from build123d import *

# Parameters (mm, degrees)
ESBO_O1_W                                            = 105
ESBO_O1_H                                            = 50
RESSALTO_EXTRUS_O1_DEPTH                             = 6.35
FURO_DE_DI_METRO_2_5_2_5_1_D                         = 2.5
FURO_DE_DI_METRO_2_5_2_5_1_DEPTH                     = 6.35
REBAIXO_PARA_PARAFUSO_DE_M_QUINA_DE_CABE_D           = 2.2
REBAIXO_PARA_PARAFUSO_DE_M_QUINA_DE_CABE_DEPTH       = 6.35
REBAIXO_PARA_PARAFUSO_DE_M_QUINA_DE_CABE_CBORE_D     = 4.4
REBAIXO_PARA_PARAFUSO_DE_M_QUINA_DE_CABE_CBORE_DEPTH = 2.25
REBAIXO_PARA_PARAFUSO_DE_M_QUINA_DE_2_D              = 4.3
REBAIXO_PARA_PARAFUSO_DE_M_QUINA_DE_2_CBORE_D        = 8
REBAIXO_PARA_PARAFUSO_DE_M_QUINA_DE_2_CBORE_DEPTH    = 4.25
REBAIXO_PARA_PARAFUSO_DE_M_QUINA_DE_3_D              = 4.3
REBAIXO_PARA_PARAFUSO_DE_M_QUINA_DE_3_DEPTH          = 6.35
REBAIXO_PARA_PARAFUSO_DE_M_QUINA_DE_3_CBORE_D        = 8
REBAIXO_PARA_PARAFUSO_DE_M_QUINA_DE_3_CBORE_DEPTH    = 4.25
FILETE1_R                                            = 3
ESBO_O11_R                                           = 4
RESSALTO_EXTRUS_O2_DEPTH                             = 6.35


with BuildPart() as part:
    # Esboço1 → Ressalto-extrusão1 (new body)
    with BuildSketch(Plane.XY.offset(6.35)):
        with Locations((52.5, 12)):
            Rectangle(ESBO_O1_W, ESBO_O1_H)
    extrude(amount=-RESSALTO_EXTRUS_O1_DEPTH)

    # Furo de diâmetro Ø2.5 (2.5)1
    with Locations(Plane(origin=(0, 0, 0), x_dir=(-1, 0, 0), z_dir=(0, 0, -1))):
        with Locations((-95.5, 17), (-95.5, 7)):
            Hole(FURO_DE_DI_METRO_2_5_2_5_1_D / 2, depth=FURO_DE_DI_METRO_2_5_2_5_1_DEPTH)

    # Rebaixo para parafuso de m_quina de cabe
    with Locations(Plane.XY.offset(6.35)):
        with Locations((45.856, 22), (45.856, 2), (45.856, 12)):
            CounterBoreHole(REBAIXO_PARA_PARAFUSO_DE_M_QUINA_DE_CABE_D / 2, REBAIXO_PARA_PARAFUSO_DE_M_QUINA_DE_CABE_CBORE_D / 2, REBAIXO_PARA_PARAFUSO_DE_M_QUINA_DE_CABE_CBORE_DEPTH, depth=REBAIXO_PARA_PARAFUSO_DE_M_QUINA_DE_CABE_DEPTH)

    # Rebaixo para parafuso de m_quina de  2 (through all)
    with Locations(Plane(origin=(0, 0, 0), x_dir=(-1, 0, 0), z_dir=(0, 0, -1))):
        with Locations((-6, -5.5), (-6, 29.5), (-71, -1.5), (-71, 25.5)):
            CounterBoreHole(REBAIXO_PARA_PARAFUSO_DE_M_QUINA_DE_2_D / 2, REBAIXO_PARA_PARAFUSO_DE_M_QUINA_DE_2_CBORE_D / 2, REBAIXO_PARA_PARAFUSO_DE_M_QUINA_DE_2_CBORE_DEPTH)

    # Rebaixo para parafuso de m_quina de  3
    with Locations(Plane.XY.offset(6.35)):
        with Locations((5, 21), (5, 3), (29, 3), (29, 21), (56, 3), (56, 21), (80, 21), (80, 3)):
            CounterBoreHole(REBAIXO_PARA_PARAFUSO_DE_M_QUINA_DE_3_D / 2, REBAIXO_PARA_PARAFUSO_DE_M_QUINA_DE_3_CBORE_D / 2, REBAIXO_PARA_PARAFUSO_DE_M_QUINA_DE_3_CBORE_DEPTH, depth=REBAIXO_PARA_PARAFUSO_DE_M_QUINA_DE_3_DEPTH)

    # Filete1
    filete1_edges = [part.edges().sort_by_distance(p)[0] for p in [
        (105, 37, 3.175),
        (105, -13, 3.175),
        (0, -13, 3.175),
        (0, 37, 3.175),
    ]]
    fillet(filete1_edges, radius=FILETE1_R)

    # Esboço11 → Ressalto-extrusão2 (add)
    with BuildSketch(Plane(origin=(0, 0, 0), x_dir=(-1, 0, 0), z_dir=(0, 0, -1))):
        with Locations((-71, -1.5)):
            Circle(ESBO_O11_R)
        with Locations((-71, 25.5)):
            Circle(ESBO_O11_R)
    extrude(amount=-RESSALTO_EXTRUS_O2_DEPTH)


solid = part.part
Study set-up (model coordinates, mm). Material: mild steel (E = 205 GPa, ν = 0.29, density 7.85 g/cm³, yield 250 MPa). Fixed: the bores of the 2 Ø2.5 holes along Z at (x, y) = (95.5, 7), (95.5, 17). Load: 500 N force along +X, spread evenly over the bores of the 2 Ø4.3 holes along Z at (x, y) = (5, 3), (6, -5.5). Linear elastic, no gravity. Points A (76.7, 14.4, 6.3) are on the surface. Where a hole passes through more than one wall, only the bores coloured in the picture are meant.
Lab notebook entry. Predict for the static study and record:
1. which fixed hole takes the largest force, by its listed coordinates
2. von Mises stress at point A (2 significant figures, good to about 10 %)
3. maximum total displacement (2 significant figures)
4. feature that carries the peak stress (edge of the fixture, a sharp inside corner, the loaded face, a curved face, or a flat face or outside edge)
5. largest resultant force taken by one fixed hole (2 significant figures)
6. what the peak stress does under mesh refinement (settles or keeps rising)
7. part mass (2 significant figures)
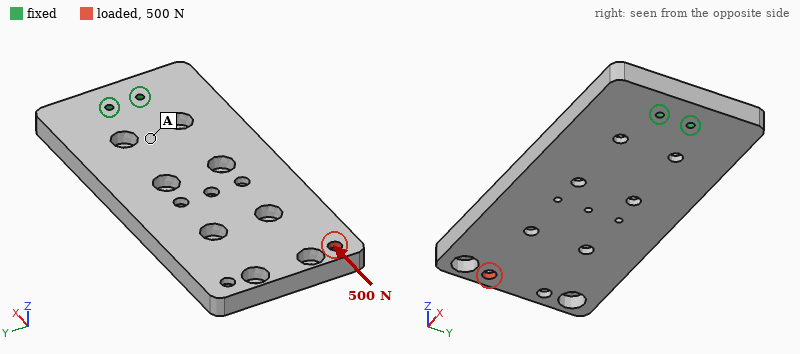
(95.5, 7)
2.6 MPa
8.9 µm
edge of the fixture
810 N
keeps rising
240 g
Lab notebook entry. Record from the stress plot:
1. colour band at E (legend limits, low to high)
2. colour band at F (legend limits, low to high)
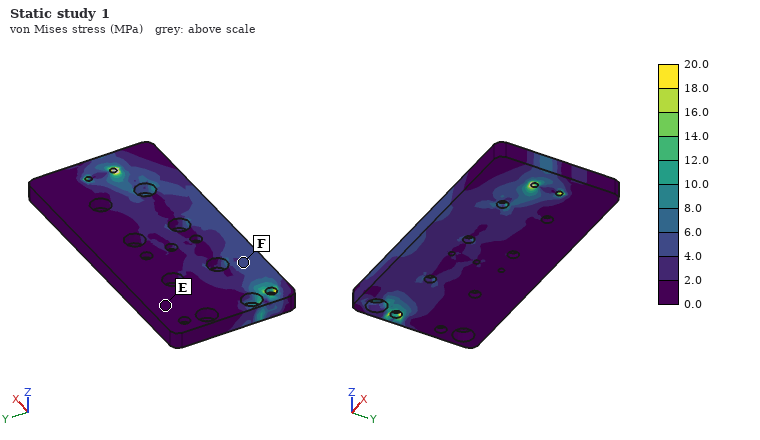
0.0 to 2.0 MPa
4.0 to 6.0 MPa
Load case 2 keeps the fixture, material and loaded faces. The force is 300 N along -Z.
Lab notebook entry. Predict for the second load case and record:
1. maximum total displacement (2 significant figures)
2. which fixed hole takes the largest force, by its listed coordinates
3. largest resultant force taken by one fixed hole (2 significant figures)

0.50 mm
(95.5, 7)
360 N
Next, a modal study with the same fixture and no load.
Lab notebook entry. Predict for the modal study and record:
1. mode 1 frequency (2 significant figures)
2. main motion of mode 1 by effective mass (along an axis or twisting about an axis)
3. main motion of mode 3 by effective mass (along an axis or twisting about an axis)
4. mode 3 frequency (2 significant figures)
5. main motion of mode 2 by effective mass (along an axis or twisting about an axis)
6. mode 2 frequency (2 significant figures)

540 Hz
along Z
twisting about X
2000 Hz
along Y
1800 Hz
